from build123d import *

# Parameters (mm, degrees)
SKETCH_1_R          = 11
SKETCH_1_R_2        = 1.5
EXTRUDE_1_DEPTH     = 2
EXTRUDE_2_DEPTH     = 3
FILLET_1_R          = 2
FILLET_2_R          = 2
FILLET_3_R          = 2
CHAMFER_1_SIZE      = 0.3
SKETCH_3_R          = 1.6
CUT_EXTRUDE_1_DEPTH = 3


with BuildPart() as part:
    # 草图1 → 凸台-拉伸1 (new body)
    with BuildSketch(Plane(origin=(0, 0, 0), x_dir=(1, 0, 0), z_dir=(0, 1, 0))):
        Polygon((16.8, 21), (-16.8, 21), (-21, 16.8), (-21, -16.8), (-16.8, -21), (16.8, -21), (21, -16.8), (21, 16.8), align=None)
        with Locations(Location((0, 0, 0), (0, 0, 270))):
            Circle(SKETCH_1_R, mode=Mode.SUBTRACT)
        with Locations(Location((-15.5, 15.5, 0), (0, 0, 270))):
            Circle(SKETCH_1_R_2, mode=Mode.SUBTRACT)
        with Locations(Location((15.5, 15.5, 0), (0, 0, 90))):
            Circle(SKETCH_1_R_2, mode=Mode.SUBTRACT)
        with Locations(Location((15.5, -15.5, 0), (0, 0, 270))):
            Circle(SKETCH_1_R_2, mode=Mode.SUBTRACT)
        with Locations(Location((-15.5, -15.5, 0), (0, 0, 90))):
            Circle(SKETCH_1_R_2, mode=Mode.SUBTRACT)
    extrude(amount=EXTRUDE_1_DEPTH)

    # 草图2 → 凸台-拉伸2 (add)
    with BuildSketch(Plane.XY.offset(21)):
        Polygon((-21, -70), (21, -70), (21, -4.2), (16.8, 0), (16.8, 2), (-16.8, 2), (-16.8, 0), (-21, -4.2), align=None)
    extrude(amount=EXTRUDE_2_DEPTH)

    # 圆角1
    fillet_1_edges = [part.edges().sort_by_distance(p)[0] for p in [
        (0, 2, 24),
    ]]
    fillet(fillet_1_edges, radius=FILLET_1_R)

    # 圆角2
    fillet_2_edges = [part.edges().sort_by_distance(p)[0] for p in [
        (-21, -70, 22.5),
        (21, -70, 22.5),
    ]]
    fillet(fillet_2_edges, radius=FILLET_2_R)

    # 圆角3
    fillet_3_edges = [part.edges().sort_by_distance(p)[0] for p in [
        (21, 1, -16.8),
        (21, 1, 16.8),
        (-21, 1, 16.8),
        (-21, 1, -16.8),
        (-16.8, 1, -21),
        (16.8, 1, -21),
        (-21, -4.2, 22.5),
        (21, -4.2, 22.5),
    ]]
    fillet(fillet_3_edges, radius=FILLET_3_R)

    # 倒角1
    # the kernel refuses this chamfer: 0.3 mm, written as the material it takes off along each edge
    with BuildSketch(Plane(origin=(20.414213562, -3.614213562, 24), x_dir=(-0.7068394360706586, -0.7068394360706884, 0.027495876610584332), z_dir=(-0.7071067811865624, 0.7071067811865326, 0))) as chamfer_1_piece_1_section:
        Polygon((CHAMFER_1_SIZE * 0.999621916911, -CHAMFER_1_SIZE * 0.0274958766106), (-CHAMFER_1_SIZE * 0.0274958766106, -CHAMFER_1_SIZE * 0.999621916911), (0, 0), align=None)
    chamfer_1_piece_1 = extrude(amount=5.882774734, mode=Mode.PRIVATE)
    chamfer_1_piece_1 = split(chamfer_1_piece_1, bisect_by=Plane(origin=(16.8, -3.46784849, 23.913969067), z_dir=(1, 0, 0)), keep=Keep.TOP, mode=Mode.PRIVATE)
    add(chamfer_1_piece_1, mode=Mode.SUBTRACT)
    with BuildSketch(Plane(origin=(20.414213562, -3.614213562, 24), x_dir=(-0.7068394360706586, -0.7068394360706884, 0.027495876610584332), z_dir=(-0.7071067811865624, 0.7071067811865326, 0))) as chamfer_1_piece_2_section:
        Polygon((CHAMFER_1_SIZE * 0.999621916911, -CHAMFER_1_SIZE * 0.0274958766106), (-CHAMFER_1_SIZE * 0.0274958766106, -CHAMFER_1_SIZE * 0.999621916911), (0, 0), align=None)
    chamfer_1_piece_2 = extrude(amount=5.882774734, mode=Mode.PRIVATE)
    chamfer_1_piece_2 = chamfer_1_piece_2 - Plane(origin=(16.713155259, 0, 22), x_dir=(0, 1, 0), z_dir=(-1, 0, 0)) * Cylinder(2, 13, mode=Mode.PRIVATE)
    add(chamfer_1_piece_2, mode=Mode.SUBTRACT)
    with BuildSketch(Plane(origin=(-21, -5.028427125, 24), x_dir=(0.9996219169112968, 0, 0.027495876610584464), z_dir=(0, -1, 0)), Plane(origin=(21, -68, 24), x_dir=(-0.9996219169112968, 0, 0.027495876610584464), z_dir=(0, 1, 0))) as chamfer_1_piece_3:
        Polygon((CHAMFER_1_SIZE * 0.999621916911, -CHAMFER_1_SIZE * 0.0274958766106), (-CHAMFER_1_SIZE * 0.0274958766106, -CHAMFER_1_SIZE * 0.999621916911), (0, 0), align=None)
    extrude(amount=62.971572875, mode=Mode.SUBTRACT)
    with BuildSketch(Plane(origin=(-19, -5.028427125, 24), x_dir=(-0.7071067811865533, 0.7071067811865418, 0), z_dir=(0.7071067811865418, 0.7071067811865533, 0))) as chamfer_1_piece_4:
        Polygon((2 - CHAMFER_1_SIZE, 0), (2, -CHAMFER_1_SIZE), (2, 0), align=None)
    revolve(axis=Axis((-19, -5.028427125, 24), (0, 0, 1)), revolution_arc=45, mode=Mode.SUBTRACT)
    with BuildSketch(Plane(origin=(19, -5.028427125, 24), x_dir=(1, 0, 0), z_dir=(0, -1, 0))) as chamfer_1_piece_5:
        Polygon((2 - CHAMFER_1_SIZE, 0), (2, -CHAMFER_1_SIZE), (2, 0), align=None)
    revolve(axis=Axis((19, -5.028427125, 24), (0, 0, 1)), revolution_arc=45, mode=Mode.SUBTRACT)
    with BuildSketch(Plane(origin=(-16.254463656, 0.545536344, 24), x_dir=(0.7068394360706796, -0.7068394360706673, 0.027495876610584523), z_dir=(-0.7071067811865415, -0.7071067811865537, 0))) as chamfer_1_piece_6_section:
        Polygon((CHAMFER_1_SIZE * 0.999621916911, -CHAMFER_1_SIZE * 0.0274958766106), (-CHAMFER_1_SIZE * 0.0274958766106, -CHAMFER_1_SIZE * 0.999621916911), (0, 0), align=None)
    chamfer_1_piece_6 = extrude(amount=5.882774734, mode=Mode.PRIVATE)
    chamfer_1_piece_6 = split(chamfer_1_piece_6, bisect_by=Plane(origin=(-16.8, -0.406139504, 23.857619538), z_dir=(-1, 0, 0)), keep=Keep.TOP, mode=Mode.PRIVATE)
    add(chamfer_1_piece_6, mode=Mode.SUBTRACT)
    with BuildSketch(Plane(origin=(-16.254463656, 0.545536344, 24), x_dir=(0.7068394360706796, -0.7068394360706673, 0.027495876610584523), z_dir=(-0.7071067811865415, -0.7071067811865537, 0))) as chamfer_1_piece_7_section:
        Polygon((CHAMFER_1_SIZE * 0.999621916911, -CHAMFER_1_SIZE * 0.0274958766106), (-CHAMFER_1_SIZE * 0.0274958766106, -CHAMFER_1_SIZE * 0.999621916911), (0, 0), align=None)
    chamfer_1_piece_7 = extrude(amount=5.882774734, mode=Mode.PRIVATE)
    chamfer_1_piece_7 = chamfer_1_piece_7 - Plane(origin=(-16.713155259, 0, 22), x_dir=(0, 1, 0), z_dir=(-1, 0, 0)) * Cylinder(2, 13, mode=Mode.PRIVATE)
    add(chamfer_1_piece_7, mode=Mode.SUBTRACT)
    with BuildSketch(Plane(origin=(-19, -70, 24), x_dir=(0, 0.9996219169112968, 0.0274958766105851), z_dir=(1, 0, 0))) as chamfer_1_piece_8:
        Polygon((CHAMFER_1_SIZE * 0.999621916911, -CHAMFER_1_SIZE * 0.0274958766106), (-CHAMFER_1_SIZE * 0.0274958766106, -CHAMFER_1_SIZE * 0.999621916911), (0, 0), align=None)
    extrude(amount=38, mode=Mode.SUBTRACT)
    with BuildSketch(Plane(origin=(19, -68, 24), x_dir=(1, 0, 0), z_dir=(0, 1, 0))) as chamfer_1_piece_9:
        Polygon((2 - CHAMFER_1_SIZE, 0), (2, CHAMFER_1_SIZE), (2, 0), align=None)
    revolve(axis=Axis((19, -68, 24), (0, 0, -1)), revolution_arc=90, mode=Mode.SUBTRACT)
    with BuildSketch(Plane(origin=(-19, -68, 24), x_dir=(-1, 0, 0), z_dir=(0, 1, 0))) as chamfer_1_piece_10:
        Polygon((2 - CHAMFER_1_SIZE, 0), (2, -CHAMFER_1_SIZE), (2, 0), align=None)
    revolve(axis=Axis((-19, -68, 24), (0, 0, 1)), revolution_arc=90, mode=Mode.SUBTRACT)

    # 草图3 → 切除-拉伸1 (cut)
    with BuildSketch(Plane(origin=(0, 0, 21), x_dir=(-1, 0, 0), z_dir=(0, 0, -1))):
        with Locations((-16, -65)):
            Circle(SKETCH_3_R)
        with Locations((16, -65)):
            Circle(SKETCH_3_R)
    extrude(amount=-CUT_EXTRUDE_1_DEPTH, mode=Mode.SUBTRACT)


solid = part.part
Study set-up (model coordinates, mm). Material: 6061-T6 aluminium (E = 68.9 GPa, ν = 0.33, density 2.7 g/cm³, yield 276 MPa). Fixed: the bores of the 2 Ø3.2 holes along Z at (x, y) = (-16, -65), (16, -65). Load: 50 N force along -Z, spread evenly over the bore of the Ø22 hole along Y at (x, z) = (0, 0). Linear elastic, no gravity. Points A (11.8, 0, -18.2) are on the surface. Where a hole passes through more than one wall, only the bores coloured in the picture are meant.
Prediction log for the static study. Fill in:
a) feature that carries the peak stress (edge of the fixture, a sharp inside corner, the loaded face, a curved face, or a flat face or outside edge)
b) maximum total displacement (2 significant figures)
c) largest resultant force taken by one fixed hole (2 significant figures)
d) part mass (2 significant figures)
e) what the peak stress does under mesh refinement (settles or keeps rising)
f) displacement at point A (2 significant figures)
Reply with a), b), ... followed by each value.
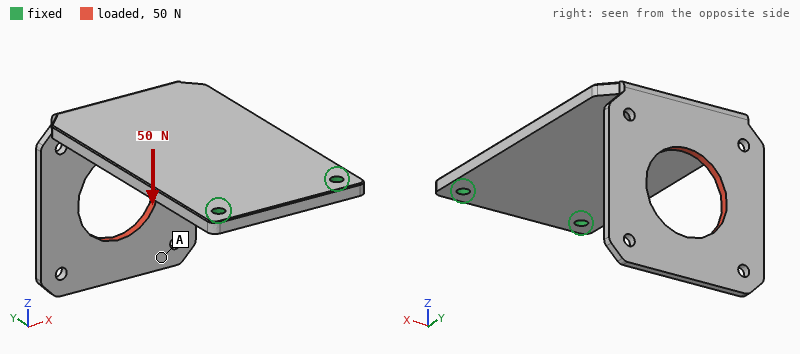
a) edge of the fixture
b) 1.1 mm
c) 25 N
d) 31 g
e) keeps rising
f) 1.1 mm
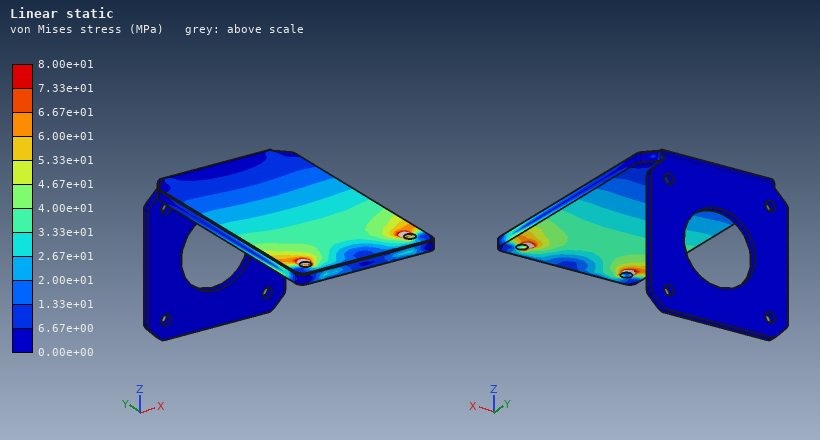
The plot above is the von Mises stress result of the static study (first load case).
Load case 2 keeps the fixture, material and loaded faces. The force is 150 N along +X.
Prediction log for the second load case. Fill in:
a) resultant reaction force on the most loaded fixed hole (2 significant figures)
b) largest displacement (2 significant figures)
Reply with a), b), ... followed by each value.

a) 330 N
b) 0.94 mm
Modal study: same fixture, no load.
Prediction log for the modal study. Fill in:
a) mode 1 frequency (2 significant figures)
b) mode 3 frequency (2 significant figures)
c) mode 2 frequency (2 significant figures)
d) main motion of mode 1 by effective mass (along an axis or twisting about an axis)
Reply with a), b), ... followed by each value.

a) 320 Hz
b) 780 Hz
c) 760 Hz
d) along Z
